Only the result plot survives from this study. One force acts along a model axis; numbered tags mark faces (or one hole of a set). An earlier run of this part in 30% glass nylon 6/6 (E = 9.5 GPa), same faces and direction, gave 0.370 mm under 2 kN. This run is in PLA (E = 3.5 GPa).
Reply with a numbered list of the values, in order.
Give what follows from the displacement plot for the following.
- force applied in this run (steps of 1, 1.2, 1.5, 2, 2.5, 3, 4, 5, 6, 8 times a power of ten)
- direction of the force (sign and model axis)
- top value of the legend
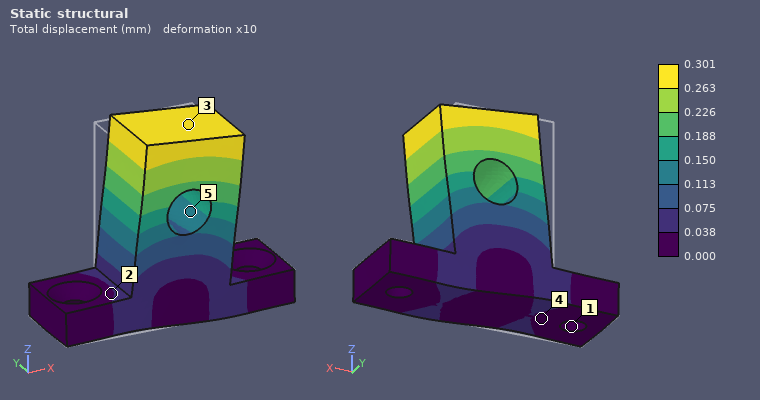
1. 600 N
2. +X
3. 0.301 mm
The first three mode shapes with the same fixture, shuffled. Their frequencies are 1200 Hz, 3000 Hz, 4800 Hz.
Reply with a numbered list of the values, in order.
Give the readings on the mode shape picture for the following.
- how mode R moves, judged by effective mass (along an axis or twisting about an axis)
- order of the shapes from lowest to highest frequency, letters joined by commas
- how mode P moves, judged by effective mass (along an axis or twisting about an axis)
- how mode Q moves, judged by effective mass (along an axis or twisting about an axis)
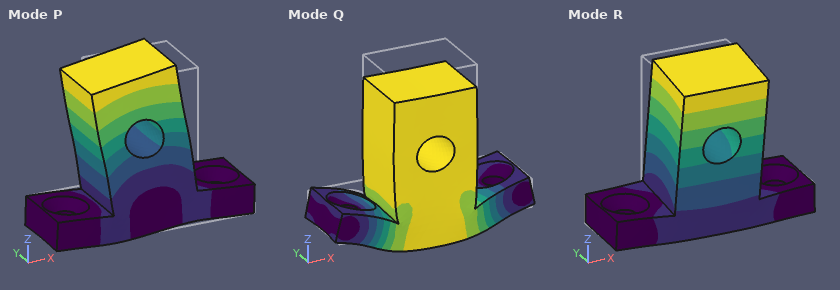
1. along Y
2. R, P, Q
3. along X
4. along Z
